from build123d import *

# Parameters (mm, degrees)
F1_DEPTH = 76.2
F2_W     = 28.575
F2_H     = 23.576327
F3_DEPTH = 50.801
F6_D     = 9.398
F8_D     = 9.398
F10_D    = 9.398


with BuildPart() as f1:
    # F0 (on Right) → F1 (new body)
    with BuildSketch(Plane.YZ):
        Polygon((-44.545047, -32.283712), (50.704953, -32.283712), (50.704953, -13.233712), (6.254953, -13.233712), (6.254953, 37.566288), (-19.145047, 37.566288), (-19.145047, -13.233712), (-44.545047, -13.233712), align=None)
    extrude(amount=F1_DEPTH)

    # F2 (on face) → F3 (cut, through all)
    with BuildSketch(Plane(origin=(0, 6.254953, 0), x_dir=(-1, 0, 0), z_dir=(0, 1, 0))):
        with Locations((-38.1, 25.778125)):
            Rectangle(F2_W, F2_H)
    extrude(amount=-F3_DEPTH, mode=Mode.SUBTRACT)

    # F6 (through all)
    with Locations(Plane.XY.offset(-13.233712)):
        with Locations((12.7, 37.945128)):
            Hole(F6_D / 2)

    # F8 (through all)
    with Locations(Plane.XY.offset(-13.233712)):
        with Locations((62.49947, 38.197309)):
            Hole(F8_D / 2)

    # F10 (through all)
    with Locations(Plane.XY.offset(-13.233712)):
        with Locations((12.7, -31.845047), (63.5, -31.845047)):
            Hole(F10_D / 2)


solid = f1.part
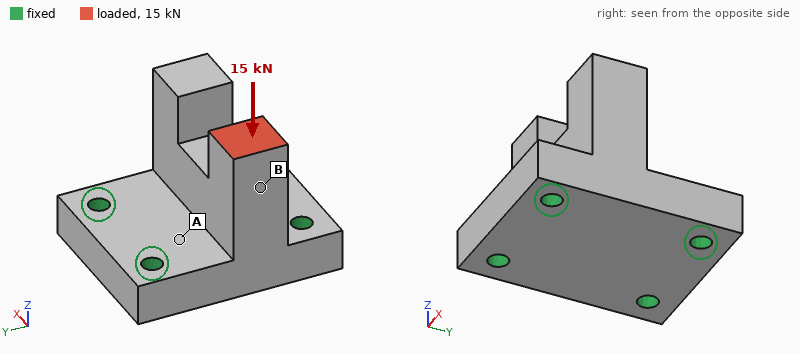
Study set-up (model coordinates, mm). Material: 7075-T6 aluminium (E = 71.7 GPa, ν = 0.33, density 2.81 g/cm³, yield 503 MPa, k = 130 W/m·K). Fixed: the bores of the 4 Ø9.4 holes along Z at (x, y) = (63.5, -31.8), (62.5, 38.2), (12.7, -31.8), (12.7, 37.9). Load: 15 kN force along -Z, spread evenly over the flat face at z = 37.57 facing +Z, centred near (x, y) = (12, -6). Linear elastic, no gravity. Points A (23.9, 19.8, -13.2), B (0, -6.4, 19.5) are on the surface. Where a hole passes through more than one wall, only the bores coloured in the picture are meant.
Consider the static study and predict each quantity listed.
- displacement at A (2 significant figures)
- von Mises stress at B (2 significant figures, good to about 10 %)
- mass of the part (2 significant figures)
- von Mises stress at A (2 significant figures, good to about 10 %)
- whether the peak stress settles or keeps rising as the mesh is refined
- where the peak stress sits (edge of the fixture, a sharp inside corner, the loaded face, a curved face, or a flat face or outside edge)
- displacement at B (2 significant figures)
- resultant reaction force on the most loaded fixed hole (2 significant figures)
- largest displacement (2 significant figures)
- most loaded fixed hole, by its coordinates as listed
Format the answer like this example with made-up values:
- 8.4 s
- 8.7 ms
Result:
- 9.4 µm
- 26 MPa
- 600 g
- 9.9 MPa
- keeps rising
- edge of the fixture
- 44 µm
- 9.9 kN
- 58 µm
- (12.7, -31.8)
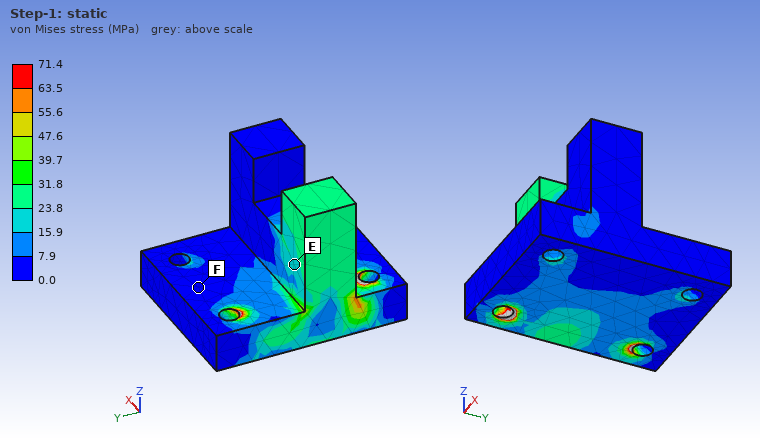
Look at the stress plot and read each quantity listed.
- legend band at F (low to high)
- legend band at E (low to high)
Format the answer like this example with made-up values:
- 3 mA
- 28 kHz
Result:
- 0.0 to 7.9 MPa
- 15.9 to 23.8 MPa
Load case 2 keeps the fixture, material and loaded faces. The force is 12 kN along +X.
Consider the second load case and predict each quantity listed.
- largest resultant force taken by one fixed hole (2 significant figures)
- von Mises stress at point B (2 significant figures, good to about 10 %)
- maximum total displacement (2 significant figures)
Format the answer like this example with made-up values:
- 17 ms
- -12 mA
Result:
- 11 kN
- 86 MPa
- 0.19 mm
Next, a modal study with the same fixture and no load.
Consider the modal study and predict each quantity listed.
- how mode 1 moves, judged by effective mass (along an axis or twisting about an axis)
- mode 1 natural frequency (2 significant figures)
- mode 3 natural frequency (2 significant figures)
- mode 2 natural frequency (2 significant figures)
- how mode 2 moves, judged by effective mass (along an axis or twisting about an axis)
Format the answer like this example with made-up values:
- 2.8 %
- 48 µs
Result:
- along Y
- 5500 Hz
- 7300 Hz
- 6200 Hz
- along X
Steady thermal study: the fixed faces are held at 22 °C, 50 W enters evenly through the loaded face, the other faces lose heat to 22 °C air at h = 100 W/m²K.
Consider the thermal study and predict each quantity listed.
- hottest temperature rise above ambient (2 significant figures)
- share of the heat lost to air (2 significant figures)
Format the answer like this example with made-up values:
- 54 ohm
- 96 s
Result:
- 29 K
- 23 %
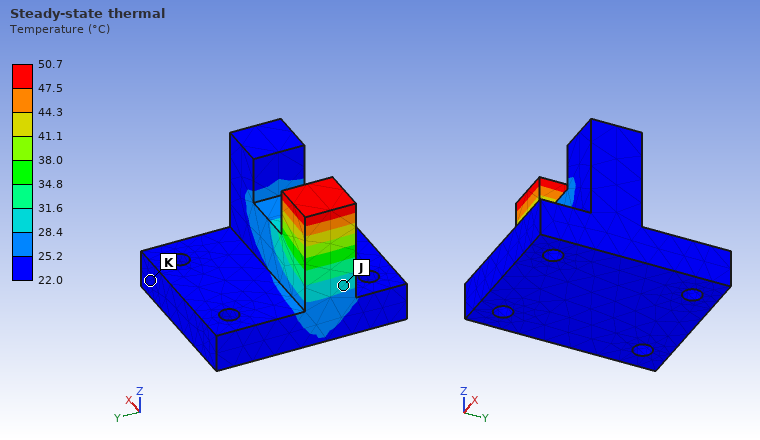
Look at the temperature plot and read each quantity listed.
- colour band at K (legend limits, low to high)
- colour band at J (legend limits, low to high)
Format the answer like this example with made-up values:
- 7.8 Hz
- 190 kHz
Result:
- 22.0 to 25.2 °C
- 28.4 to 31.6 °C
